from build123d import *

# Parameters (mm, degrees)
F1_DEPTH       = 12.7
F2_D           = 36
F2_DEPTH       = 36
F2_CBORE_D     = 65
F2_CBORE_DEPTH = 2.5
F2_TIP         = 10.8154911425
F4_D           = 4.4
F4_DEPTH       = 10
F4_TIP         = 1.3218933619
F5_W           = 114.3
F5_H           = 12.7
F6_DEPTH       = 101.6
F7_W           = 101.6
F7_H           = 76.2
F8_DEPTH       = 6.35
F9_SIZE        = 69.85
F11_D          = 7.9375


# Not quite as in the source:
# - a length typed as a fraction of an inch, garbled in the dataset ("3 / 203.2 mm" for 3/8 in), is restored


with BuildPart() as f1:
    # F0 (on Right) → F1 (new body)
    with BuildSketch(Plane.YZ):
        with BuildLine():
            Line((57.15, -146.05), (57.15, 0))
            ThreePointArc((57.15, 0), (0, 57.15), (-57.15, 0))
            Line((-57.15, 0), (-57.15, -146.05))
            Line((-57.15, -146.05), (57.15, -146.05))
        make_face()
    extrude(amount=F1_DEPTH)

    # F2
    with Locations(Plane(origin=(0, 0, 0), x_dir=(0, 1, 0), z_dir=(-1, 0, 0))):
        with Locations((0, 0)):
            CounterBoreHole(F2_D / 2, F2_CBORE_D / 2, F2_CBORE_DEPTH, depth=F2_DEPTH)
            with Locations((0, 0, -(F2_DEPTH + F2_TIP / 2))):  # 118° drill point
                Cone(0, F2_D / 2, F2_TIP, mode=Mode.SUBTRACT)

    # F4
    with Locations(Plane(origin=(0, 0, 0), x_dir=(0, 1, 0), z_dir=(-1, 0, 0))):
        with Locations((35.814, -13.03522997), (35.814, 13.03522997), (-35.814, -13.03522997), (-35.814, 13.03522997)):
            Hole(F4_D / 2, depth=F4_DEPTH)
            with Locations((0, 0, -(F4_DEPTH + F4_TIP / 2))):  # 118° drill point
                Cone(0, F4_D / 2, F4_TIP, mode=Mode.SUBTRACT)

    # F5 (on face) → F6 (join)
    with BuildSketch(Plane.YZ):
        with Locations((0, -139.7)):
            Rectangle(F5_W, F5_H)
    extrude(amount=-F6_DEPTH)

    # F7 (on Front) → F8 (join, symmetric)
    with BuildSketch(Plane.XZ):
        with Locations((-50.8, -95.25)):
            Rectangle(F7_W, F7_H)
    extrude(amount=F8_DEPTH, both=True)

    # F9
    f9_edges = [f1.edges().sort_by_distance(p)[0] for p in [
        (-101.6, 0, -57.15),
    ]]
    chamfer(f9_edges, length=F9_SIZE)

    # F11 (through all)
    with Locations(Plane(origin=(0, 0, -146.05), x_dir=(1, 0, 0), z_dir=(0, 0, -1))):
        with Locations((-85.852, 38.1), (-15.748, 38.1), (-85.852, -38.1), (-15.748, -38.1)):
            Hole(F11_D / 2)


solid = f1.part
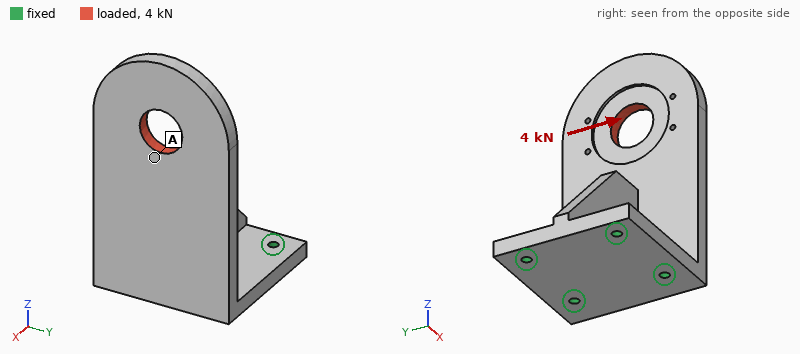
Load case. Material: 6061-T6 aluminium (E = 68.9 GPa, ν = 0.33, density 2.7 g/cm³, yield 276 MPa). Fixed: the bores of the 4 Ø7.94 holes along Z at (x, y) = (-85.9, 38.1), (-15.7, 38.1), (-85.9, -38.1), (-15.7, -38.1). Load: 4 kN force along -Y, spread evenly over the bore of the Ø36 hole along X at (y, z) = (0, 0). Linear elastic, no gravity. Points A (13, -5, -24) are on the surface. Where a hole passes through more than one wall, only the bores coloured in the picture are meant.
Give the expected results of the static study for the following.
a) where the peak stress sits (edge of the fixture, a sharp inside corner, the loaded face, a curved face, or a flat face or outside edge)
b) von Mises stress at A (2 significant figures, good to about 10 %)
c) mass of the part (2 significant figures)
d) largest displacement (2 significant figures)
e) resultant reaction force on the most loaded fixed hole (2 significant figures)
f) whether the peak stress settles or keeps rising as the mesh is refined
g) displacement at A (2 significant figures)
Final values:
edge of the fixture
12 MPa
1.3 kg
0.25 mm
7.3 kN
keeps rising
0.14 mm
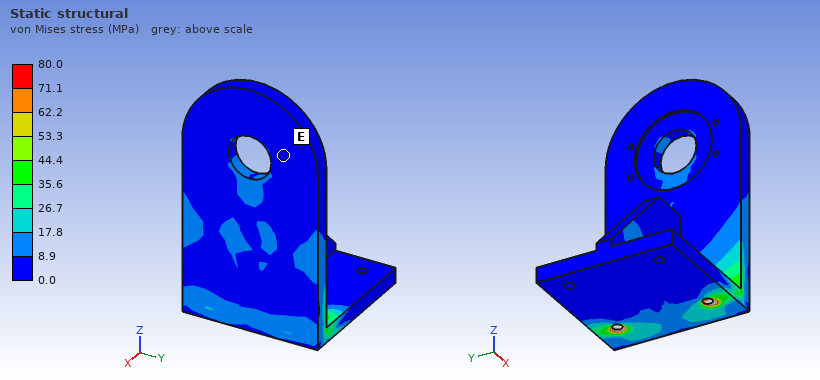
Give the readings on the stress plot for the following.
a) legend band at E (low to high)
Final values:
0.0 to 8.9 MPa
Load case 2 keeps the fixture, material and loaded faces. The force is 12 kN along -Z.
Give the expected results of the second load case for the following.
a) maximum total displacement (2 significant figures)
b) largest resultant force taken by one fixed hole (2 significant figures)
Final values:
0.20 mm
7.2 kN
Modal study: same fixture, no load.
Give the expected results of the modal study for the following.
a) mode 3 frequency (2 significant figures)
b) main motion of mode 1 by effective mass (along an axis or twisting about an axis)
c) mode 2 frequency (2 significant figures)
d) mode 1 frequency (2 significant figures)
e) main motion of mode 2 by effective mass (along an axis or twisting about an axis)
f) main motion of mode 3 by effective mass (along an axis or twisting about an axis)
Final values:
1300 Hz
along X
1100 Hz
640 Hz
along Y
along Y
